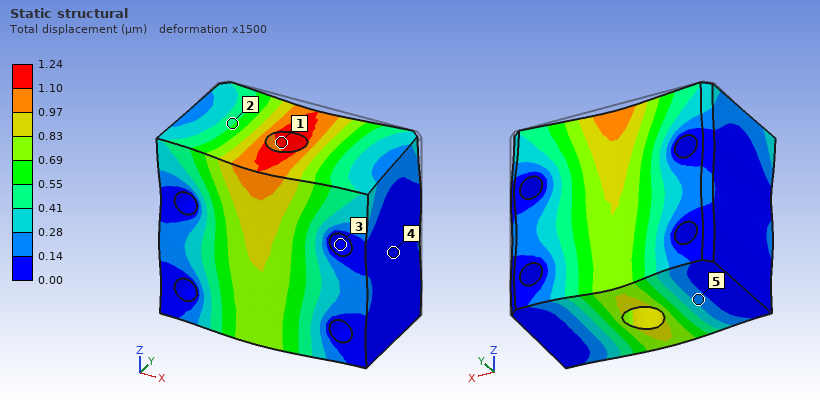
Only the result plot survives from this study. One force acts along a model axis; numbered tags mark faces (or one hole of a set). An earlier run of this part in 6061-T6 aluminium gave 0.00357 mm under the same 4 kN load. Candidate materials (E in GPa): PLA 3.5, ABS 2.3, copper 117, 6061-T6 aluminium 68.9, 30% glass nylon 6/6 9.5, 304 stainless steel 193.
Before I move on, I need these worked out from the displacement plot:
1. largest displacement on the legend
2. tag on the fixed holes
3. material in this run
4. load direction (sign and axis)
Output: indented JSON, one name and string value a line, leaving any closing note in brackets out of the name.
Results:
{
  "largest displacement on the legend": "1.24 µm",
  "tag on the fixed holes": "3",
  "material in this run": "304 stainless steel",
  "load direction": "-Y"
}
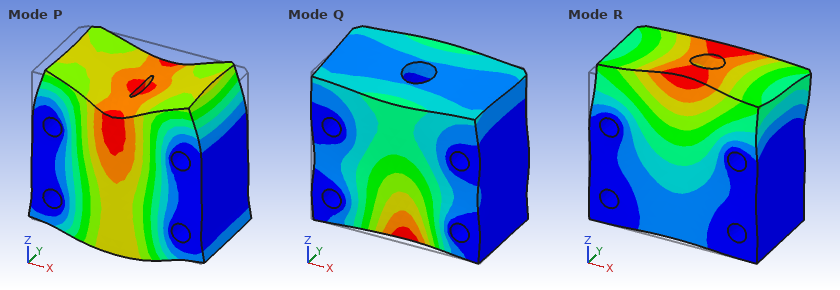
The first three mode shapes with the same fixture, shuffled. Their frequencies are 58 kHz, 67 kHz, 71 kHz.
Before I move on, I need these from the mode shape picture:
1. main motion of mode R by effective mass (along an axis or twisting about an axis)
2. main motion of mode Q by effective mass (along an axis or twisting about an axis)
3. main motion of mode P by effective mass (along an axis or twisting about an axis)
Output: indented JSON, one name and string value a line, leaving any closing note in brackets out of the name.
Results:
{
  "main motion of mode R by effective mass": "along Y",
  "main motion of mode Q by effective mass": "along Y",
  "main motion of mode P by effective mass": "along Z"
}
